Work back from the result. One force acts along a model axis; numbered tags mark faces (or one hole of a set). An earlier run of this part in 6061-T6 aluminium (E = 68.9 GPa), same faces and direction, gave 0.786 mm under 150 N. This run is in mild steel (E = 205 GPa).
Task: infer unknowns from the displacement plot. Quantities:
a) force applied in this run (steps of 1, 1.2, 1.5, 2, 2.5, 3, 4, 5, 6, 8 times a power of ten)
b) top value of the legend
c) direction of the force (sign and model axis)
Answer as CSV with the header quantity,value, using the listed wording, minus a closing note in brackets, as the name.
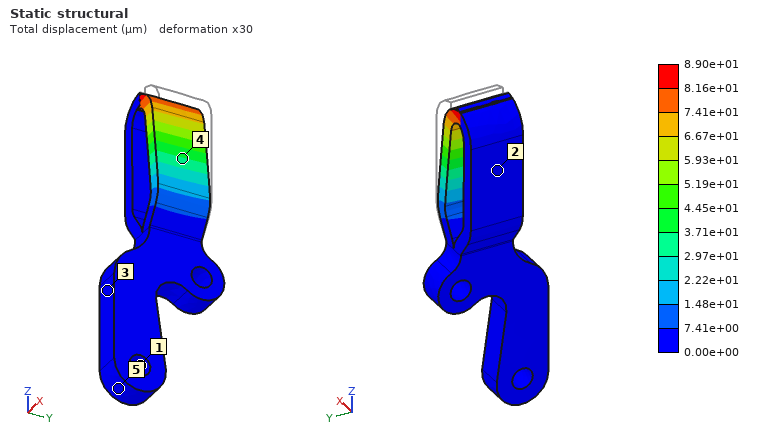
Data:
quantity,value
force applied in this run,50 N
top value of the legend,8.90e+01 µm
direction of the force,-X
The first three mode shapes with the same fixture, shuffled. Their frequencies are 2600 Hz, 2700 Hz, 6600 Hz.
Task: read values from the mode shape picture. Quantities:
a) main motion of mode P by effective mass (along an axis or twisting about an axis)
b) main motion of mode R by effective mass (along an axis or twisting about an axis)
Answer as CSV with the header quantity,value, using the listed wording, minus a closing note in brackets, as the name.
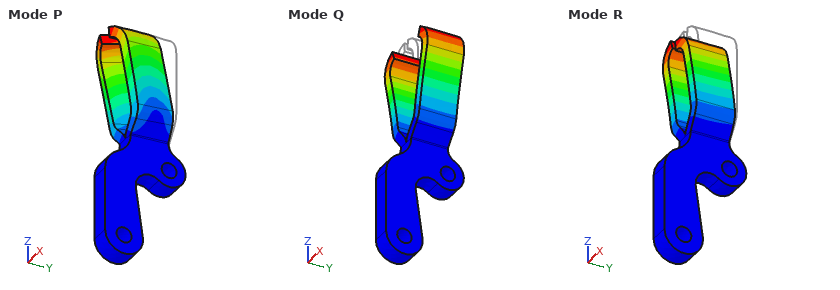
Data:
quantity,value
main motion of mode P by effective mass,along Y
main motion of mode R by effective mass,along X
